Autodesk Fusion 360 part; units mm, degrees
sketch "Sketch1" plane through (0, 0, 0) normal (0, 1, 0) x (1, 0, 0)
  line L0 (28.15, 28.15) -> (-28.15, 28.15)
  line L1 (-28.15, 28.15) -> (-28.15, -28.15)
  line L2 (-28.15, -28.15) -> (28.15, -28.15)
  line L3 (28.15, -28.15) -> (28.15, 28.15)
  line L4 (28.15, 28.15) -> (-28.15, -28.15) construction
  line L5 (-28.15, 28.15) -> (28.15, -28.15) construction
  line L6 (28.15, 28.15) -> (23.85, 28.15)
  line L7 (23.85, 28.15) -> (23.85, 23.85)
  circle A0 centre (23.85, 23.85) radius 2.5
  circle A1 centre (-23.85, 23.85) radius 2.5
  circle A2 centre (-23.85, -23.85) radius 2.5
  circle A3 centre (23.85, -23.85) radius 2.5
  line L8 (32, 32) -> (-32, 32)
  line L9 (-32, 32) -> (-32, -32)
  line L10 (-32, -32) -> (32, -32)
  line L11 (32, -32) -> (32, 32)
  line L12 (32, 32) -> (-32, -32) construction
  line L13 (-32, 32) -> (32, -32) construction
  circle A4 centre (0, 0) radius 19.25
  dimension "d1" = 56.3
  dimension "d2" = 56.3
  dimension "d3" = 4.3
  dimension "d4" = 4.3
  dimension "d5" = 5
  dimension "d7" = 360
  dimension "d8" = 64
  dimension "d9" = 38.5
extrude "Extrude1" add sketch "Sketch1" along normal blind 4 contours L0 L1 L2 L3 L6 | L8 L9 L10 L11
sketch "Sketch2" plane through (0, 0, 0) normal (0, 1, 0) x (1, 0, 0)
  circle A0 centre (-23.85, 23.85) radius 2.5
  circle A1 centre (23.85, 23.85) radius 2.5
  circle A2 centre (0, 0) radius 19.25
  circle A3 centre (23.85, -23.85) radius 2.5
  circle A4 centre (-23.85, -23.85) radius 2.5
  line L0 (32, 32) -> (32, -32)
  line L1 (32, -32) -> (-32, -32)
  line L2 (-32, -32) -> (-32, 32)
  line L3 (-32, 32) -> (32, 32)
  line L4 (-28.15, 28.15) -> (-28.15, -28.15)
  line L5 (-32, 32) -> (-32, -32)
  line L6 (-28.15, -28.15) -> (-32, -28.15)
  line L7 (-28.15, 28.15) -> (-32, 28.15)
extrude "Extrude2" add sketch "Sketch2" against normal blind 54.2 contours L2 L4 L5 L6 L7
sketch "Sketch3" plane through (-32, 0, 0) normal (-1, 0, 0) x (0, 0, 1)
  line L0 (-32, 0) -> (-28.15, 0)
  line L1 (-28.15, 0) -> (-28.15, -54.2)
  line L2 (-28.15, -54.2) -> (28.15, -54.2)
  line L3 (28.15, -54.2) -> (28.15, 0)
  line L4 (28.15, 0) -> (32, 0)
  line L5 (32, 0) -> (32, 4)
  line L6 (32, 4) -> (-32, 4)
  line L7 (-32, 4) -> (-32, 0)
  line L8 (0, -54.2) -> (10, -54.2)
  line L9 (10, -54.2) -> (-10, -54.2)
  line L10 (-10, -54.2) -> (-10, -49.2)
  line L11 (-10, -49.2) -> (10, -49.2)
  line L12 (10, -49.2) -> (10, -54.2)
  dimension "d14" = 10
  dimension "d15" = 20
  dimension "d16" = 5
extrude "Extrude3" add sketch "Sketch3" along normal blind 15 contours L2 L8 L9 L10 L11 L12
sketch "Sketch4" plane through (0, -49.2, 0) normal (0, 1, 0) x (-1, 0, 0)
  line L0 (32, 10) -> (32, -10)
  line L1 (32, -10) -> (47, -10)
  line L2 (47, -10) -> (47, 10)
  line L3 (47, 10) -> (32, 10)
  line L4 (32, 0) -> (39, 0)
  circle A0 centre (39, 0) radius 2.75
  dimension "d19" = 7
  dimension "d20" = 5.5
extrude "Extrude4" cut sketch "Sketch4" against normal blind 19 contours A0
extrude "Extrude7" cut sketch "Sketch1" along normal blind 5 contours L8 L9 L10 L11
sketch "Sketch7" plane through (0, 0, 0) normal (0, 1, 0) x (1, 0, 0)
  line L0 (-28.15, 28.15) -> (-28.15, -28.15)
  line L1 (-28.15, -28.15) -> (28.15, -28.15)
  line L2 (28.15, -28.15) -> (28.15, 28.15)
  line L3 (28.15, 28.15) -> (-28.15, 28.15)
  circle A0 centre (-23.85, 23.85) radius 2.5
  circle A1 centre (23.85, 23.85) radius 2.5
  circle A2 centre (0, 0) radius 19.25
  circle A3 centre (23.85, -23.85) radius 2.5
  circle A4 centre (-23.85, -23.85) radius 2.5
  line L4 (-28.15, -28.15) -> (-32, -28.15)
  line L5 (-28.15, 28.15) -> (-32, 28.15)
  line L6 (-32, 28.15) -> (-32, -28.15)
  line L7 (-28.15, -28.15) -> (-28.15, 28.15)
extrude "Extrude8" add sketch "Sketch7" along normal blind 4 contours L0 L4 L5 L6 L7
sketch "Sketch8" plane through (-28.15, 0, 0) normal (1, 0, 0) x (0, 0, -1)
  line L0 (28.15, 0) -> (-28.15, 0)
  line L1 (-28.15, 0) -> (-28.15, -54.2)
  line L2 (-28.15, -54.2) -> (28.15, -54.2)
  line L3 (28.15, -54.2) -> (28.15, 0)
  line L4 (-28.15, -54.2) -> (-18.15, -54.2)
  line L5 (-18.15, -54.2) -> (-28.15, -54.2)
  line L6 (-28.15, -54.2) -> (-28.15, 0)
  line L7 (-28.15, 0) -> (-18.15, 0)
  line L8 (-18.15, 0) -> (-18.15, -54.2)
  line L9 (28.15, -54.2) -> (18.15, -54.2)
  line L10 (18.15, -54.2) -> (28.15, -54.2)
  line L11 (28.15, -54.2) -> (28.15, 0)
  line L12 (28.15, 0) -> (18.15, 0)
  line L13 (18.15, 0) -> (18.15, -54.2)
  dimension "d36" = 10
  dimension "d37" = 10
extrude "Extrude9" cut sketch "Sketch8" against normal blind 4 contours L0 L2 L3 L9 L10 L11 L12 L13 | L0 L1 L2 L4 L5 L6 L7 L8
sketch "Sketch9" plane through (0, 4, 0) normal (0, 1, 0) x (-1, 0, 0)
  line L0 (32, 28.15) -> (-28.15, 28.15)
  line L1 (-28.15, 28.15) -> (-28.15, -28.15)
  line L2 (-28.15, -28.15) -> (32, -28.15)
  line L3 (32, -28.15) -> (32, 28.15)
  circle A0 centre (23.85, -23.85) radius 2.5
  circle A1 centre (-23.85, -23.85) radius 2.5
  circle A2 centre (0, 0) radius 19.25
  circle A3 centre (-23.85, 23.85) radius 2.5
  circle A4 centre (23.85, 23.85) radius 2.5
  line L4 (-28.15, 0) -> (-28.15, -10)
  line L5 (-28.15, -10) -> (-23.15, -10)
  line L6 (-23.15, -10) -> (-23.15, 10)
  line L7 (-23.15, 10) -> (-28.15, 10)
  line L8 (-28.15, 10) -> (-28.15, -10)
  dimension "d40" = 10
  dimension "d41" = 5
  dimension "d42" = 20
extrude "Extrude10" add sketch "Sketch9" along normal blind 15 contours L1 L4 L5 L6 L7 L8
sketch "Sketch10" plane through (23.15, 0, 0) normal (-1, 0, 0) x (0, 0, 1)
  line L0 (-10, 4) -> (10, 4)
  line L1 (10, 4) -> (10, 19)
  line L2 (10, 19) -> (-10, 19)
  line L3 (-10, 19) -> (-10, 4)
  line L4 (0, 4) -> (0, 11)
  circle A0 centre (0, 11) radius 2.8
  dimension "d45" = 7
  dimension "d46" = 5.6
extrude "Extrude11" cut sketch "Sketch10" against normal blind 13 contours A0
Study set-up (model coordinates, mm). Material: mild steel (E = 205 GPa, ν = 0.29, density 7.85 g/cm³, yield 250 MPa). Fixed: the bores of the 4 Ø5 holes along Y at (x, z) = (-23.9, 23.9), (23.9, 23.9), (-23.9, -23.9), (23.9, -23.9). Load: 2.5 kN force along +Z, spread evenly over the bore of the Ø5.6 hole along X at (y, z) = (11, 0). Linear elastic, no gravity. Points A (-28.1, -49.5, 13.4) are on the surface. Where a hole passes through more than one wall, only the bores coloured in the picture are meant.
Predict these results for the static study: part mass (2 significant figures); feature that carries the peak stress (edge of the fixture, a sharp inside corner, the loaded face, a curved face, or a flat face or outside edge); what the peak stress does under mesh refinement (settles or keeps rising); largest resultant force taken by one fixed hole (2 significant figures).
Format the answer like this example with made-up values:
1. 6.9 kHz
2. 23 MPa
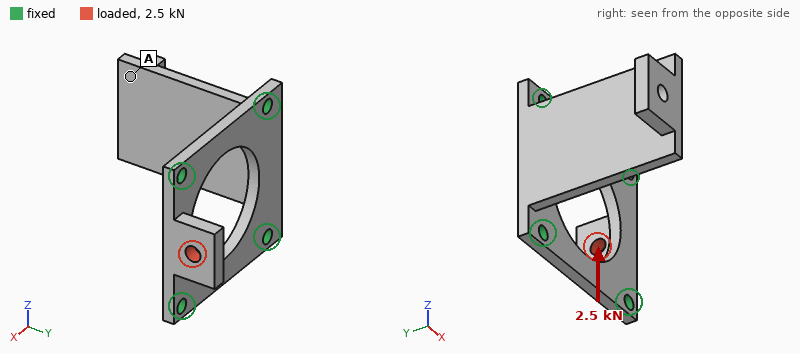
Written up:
1. 150 g
2. edge of the fixture
3. keeps rising
4. 1.4 kN
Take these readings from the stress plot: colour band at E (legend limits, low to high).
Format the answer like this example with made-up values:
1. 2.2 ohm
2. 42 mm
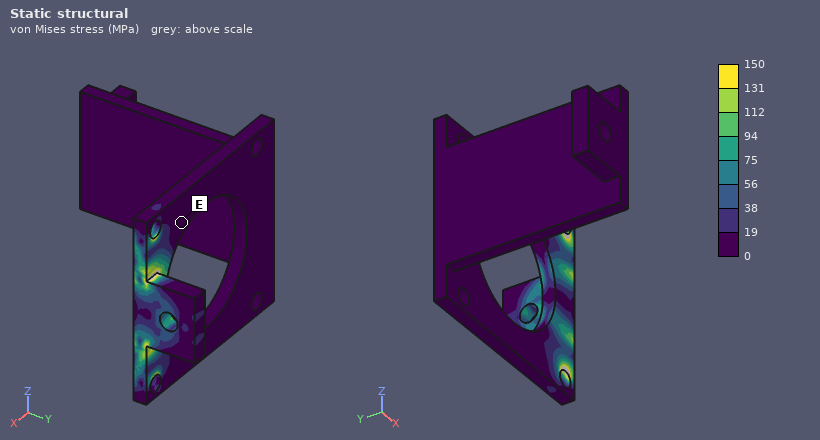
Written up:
1. 0 to 19 MPa
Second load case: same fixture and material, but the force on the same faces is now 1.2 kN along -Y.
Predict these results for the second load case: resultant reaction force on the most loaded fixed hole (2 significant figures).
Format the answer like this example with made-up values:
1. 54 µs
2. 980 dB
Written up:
1. 670 N
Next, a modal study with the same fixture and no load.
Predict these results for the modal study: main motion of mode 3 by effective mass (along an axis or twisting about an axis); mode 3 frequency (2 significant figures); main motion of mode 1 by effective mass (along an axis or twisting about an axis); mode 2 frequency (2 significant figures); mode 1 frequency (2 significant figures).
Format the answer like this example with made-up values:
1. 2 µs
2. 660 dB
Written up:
1. along Z
2. 3600 Hz
3. along X
4. 2700 Hz
5. 650 Hz
